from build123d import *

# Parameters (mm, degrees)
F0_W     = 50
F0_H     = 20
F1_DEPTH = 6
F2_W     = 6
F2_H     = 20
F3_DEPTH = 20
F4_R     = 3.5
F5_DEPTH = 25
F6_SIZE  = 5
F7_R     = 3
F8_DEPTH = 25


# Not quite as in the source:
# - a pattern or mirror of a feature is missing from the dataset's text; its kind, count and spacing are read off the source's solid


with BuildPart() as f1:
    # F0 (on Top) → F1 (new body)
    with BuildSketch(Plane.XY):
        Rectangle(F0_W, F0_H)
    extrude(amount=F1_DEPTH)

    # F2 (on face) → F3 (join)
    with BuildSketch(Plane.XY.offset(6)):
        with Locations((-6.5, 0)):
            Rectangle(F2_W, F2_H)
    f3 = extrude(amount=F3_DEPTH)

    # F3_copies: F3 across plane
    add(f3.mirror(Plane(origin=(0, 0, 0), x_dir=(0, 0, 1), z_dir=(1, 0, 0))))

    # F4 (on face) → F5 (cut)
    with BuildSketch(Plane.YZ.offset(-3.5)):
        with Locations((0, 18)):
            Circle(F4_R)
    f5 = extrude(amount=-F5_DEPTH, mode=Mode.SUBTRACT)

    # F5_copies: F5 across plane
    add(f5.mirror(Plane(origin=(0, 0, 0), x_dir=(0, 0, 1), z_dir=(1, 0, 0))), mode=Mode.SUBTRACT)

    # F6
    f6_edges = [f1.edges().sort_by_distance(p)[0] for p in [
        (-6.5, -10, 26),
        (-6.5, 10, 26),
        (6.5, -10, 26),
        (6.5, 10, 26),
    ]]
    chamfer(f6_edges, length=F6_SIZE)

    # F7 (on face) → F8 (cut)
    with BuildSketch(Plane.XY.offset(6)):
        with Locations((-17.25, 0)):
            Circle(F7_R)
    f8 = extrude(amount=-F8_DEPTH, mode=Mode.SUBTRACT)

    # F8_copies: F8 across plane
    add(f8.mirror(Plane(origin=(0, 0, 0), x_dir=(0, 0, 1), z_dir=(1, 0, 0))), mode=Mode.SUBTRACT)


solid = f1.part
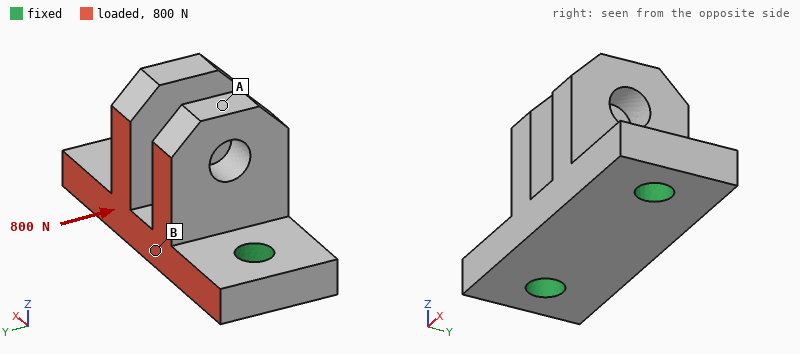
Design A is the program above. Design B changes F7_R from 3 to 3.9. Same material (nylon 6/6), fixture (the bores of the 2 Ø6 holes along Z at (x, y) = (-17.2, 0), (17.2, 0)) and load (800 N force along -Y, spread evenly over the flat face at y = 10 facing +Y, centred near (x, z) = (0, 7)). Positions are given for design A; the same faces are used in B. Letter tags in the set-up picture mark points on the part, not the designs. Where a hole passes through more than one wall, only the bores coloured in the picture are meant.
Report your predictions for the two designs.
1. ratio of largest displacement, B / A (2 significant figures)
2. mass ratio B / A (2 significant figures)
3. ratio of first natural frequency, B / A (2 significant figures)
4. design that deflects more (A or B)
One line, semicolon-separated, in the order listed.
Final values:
0.82; 0.98; 1.0; A
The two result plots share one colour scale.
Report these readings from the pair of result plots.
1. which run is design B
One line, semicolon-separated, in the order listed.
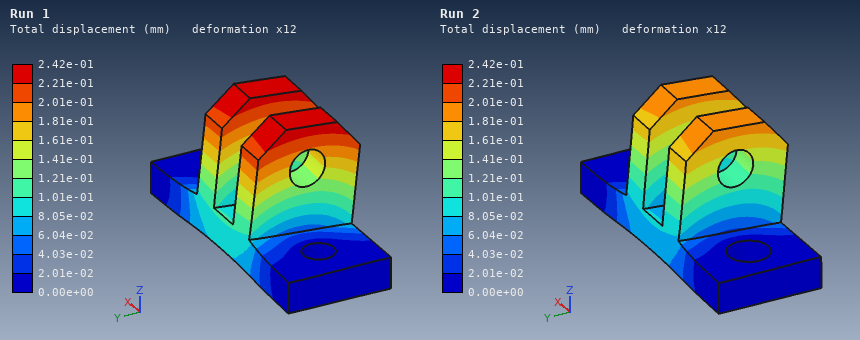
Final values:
Run 2
